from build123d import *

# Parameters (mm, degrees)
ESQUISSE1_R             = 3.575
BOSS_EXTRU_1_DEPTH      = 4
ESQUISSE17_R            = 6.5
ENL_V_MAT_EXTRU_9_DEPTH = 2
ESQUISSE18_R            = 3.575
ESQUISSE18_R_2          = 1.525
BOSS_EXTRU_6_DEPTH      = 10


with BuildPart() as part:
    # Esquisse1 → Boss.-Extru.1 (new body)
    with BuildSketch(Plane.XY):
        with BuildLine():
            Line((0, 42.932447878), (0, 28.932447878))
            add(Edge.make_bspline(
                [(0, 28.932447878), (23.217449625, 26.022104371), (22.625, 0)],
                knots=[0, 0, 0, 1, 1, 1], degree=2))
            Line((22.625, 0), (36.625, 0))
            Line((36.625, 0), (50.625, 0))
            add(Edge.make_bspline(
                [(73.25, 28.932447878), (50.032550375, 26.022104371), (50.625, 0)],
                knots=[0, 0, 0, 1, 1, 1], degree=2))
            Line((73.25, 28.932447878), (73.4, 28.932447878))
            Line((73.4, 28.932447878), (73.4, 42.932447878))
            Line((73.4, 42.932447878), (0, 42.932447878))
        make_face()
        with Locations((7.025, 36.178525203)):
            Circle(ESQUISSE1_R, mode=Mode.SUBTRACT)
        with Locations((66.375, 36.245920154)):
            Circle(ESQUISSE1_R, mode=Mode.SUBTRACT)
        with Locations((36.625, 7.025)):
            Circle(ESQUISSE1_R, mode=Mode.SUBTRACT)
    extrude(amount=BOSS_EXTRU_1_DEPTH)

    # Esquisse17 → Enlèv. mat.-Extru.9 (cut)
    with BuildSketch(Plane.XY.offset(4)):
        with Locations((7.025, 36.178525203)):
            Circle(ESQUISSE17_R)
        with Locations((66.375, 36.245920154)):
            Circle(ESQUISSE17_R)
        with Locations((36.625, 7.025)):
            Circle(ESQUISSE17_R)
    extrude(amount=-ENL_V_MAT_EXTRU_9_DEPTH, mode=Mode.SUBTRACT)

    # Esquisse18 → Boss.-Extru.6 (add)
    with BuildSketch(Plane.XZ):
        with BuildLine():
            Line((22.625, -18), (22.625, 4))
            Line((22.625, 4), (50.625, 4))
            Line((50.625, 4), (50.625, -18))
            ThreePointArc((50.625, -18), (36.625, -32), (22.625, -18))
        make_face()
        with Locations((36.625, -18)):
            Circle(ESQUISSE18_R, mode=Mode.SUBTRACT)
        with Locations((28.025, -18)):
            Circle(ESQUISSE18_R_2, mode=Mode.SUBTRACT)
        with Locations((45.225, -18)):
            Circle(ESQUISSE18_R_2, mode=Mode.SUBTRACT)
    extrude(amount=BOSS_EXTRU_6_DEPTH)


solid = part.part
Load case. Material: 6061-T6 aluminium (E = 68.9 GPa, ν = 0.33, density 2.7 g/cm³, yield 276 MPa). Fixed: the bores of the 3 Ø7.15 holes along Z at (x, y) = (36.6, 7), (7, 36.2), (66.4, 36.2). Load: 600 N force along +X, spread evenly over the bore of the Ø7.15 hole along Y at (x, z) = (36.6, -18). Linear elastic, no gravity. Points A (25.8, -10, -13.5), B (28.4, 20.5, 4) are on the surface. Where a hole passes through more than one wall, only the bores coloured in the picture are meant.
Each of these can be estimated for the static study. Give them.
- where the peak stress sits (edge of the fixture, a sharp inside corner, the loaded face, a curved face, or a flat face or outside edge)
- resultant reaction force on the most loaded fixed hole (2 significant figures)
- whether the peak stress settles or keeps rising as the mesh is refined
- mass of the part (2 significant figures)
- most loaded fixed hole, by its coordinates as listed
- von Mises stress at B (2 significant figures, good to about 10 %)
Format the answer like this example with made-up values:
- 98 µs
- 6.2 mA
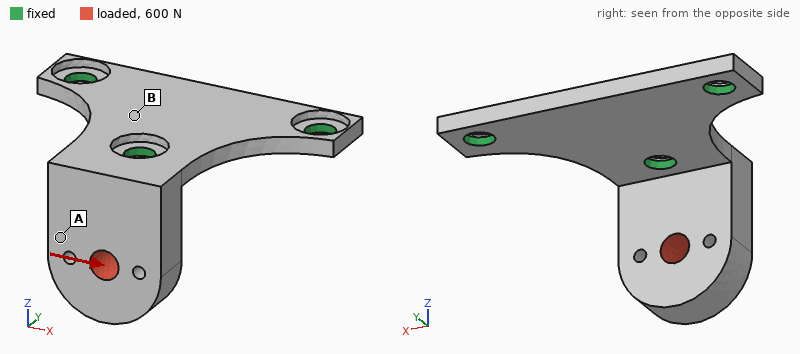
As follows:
- edge of the fixture
- 1.0 kN
- keeps rising
- 43 g
- (36.6, 7)
- 31 MPa
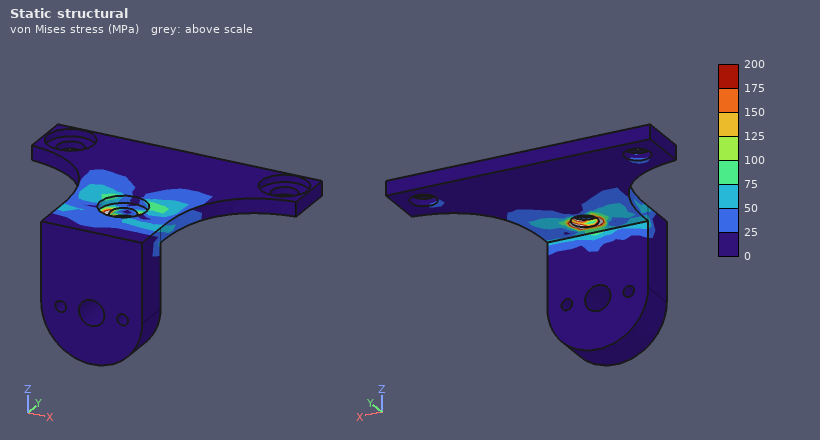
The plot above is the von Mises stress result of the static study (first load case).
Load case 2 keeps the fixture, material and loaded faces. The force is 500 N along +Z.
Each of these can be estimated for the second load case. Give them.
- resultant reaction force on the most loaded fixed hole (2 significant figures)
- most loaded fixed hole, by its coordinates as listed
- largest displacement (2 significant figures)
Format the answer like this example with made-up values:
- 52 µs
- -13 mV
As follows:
- 600 N
- (36.6, 7)
- 0.18 mm
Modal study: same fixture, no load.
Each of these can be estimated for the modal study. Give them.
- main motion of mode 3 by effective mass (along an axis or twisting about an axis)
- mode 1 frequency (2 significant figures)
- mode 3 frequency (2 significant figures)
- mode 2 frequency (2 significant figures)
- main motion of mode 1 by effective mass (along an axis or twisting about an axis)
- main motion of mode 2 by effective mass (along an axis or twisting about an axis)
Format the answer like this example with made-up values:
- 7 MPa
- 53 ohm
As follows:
- along Z
- 1500 Hz
- 6300 Hz
- 2400 Hz
- along Y
- along X
